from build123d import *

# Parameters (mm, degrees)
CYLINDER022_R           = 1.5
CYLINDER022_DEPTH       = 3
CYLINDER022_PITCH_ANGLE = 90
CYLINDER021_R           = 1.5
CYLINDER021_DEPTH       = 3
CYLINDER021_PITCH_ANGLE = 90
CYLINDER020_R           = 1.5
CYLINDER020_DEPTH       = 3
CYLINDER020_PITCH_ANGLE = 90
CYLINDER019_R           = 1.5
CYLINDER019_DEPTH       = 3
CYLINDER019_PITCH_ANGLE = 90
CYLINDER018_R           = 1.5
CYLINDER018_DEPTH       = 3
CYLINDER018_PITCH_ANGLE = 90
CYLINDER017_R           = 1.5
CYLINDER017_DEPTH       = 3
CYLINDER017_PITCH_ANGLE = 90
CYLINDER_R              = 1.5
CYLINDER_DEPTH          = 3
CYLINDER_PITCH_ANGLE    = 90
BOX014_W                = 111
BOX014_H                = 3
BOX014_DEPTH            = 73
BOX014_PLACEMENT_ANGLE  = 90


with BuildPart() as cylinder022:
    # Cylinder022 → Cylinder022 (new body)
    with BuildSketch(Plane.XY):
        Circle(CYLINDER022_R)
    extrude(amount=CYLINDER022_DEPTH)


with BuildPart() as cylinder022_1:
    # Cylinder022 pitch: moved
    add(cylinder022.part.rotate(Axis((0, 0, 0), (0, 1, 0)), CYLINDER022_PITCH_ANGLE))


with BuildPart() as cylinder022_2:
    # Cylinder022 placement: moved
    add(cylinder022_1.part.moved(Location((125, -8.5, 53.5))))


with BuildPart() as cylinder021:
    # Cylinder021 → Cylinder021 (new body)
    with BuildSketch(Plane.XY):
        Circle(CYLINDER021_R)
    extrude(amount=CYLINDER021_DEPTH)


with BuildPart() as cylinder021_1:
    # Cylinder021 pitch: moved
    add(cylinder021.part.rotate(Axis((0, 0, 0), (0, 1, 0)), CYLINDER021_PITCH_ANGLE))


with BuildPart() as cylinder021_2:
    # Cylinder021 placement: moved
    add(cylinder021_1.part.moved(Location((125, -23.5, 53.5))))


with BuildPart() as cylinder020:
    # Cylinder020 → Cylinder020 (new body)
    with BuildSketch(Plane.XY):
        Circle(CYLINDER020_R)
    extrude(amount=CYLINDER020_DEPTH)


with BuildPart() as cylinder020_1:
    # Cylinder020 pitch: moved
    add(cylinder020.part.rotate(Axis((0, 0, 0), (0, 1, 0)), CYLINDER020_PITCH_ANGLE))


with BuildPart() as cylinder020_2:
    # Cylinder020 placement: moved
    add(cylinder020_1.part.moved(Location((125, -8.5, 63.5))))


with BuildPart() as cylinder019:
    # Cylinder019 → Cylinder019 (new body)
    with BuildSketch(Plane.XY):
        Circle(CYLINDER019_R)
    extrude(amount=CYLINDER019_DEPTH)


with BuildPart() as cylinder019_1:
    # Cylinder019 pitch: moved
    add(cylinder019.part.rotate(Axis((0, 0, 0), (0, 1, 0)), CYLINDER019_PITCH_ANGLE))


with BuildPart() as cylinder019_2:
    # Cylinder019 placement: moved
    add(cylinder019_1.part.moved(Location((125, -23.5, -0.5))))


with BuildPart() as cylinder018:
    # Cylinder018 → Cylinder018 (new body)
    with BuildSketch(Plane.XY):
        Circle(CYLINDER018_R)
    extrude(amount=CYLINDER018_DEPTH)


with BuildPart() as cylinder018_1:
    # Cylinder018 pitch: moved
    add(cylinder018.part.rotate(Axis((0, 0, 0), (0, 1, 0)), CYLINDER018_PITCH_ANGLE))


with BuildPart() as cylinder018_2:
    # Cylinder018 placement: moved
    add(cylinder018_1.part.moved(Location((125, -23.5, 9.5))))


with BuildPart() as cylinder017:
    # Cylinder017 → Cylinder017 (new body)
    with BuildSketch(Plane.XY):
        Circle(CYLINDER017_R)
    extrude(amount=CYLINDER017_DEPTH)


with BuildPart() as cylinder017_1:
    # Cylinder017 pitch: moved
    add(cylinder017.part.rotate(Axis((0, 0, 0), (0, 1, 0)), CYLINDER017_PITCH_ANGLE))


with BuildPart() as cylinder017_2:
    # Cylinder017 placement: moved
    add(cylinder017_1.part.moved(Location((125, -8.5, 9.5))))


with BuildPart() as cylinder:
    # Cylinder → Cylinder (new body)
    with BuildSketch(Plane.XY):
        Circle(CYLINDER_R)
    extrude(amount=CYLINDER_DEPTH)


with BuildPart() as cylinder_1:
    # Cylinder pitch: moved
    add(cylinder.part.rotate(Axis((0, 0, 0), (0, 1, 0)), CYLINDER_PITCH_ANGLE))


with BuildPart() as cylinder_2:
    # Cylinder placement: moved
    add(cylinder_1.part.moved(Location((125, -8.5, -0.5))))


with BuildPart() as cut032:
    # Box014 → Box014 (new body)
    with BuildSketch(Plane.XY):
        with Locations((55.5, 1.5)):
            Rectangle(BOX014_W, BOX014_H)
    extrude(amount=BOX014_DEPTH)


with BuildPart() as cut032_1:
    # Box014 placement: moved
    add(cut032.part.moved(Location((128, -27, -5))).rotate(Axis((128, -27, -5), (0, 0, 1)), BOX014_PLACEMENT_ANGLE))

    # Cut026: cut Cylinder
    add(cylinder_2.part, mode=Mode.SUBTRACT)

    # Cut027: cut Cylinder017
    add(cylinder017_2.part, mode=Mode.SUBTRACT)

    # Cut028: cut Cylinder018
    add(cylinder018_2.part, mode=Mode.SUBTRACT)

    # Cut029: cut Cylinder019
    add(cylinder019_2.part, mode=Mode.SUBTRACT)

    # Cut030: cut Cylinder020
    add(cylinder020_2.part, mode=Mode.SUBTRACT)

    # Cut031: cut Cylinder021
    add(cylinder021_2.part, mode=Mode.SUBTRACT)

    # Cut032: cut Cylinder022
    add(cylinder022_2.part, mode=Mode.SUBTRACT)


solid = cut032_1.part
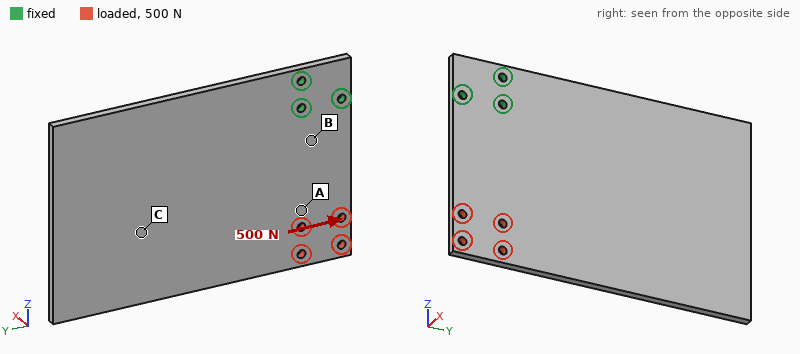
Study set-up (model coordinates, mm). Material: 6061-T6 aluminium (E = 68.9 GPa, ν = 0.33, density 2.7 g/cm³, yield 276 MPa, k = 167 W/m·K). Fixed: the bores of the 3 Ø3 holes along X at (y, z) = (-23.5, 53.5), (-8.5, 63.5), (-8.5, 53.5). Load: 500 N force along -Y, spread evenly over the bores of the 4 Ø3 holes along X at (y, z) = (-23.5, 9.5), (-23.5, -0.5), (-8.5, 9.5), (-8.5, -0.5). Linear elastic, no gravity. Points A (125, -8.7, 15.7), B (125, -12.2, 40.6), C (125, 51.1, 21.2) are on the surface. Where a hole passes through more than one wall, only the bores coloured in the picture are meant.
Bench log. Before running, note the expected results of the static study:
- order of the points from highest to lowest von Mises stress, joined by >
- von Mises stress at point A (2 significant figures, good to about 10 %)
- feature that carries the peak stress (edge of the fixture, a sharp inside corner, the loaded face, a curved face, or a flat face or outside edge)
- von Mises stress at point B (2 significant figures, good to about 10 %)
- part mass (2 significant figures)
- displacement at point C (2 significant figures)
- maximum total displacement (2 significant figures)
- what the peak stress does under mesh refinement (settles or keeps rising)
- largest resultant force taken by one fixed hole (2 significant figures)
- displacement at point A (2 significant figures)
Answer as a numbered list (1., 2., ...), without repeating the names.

1. B > A > C
2. 8.0 MPa
3. edge of the fixture
4. 18 MPa
5. 65 g
6. 57 µm
7. 91 µm
8. keeps rising
9. 1.1 kN
10. 34 µm
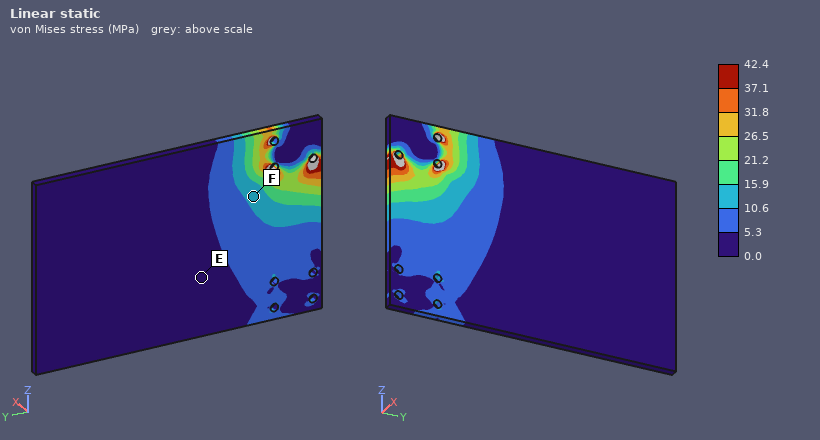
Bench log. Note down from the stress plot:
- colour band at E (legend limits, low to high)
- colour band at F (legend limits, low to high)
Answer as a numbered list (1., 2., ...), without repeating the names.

1. 0.0 to 5.3 MPa
2. 10.6 to 15.9 MPa
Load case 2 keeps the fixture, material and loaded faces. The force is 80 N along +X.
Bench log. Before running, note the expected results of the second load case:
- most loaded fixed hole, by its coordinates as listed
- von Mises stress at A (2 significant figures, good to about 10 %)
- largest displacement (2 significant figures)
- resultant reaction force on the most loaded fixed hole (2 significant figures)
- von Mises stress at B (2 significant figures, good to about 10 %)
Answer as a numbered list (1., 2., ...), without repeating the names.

1. (-8.5, 53.5)
2. 16 MPa
3. 0.59 mm
4. 200 N
5. 37 MPa
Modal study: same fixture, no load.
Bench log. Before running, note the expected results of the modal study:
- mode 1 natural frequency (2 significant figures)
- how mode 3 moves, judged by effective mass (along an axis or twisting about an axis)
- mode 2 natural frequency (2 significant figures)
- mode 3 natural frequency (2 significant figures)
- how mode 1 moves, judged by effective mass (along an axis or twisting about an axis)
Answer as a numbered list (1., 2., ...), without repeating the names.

1. 230 Hz
2. along X
3. 520 Hz
4. 1100 Hz
5. along X
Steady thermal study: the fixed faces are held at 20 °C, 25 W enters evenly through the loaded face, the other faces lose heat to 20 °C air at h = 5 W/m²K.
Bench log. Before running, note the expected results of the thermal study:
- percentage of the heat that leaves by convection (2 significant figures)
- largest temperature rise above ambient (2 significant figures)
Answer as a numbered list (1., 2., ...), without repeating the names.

1. 8.6 %
2. 67 K
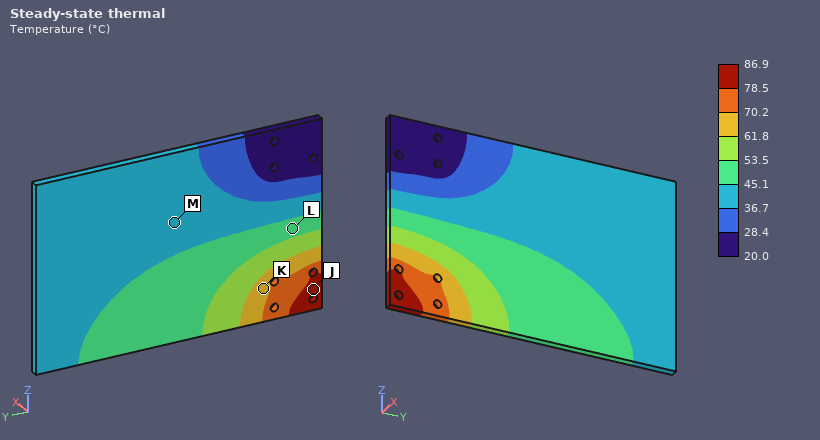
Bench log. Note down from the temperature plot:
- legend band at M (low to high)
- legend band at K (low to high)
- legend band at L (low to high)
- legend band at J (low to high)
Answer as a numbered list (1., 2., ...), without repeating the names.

1. 36.7 to 45.1 °C
2. 61.8 to 70.2 °C
3. 45.1 to 53.5 °C
4. 78.5 to 86.9 °C
